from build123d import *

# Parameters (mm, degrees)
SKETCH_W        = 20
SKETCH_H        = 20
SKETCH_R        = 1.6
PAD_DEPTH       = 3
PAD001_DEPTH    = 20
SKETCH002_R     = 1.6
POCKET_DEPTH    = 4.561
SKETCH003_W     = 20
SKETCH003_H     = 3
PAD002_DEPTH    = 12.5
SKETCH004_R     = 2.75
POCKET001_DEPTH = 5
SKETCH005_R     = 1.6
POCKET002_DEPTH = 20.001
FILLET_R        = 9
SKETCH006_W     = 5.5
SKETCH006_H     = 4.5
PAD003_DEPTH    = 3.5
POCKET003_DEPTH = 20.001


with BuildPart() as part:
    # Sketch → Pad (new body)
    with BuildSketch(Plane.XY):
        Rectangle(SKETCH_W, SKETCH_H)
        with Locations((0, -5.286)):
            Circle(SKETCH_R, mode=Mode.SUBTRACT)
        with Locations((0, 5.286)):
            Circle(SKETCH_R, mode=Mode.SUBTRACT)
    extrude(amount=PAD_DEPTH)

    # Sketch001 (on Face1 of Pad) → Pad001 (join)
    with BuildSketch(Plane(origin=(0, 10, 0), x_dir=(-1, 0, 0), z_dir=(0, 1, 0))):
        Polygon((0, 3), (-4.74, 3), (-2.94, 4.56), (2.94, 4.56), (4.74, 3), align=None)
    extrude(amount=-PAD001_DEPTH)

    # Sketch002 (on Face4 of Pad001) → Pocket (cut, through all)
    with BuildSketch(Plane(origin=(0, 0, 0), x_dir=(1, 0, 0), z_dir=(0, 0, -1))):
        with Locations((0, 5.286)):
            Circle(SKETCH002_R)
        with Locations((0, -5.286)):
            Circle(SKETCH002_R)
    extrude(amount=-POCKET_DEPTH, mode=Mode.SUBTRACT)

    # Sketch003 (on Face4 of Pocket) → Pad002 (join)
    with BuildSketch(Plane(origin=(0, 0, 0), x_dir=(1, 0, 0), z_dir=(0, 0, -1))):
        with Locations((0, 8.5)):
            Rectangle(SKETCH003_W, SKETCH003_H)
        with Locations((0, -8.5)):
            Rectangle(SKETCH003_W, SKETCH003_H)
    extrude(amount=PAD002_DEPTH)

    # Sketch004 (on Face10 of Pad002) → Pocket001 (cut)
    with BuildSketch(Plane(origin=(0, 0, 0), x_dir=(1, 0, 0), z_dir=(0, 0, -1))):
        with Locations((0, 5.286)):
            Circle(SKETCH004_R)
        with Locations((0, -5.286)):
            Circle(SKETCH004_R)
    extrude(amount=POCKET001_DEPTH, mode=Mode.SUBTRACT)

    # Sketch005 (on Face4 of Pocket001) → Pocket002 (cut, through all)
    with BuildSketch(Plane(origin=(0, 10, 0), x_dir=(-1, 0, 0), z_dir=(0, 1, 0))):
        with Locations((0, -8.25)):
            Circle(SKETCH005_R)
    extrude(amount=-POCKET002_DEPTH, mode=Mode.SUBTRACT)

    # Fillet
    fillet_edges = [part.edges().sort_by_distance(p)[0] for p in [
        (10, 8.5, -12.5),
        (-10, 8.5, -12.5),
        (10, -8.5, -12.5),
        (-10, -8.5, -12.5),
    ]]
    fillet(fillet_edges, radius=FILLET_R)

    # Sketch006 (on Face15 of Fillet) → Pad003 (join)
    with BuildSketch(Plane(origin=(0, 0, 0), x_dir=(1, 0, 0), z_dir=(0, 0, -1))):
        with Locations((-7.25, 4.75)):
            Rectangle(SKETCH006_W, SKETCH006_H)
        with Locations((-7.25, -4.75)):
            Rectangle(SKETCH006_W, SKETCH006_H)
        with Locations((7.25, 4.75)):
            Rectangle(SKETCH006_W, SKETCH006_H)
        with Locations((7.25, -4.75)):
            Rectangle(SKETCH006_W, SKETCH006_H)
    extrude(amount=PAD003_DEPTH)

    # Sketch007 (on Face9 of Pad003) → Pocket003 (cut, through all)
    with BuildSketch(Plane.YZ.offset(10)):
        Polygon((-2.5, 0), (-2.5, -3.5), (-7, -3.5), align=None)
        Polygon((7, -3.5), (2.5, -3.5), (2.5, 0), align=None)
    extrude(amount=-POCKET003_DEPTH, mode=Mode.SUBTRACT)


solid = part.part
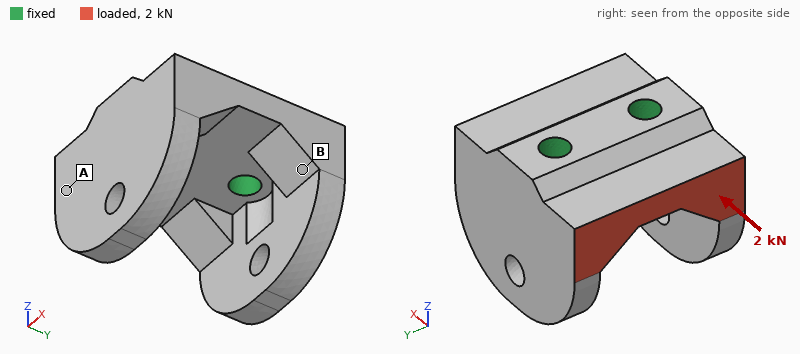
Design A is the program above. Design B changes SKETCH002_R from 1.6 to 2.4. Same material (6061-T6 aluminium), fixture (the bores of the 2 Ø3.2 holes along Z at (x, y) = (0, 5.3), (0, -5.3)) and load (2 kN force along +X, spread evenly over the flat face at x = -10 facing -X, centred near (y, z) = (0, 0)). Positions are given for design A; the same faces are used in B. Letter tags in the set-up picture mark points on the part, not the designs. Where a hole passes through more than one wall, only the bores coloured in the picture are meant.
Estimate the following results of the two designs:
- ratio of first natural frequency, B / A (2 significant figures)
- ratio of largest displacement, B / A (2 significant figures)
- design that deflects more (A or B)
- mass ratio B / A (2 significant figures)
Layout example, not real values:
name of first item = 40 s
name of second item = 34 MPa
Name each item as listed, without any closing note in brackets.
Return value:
ratio of first natural frequency, B / A = 1.1
ratio of largest displacement, B / A = 0.66
design that deflects more = A
mass ratio B / A = 0.97
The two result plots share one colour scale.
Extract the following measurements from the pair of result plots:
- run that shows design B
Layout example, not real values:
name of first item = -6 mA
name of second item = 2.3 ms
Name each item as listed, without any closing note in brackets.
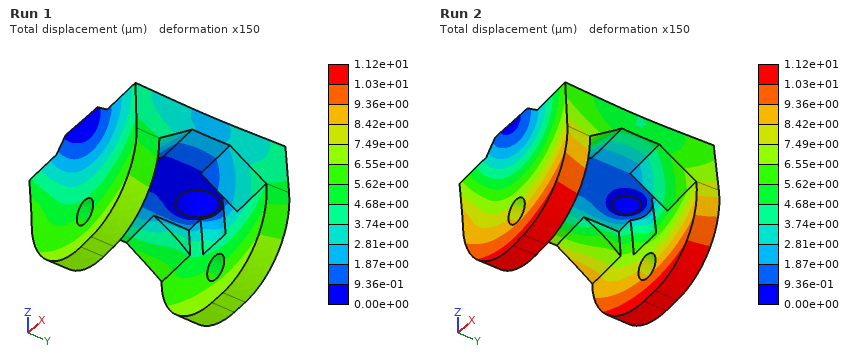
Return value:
run that shows design B = Run 1
